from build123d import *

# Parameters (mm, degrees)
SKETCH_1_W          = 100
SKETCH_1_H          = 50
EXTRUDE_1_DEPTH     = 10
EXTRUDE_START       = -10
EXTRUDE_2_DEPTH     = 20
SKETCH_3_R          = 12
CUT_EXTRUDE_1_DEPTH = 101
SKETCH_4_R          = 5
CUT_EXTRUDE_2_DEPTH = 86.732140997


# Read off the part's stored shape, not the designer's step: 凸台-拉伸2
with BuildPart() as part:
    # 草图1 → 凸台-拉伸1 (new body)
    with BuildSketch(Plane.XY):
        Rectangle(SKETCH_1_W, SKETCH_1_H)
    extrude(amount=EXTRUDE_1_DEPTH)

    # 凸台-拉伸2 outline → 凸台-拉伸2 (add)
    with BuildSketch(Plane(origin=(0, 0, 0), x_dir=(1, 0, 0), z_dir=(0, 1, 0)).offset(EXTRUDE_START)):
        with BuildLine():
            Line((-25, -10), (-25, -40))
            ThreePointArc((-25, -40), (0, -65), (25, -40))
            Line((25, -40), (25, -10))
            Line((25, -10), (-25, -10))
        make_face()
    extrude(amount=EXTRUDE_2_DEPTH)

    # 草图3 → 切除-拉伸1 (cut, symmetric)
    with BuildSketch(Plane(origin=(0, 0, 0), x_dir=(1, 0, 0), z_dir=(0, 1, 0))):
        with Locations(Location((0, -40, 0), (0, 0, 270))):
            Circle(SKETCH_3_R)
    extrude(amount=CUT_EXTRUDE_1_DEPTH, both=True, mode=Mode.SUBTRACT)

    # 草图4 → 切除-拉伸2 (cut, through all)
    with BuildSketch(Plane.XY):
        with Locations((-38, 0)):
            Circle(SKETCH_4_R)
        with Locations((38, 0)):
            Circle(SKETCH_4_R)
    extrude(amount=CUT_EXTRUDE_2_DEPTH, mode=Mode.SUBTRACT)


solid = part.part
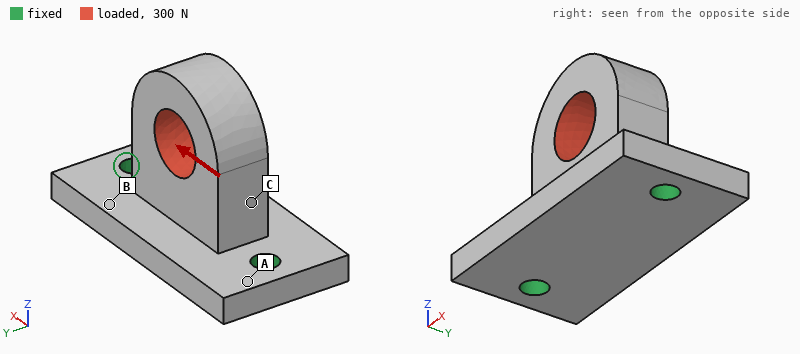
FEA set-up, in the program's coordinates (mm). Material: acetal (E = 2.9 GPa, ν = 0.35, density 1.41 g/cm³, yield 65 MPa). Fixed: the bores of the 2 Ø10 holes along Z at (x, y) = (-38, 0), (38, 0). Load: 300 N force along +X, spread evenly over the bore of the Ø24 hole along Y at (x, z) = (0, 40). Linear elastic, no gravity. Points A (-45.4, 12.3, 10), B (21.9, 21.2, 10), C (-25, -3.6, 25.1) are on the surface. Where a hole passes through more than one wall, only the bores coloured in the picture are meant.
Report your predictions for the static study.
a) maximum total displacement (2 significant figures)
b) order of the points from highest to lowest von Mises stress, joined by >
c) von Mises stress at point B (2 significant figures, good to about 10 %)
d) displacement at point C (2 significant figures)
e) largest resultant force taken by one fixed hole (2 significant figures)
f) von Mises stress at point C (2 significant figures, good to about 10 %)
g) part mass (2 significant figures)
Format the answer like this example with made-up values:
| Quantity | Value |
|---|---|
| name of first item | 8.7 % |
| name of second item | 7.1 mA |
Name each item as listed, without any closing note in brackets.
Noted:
| Quantity | Value |
|---|---|
| maximum total displacement | 67 µm |
| order of the points from highest to lowest von Mises stress, joined by > | C > B > A |
| von Mises stress at point B | 0.60 MPa |
| displacement at point C | 28 µm |
| largest resultant force taken by one fixed hole | 230 N |
| von Mises stress at point C | 1.1 MPa |
| part mass | 130 g |
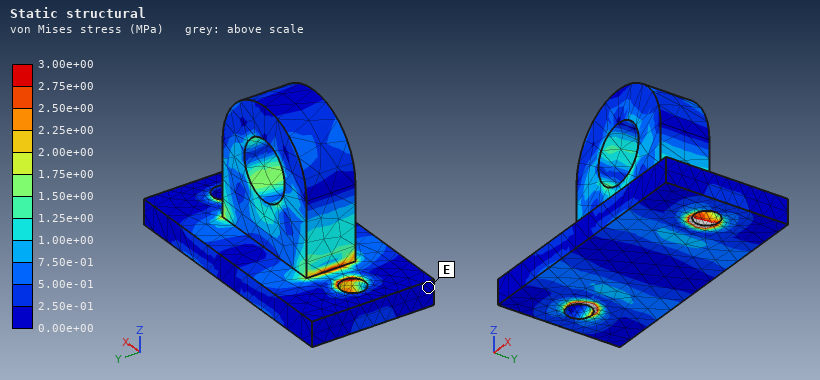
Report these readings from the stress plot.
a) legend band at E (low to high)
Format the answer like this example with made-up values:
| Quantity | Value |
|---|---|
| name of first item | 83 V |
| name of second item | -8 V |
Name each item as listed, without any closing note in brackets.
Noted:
| Quantity | Value |
|---|---|
| legend band at E | 0.00e+00 to 2.50e-01 MPa |
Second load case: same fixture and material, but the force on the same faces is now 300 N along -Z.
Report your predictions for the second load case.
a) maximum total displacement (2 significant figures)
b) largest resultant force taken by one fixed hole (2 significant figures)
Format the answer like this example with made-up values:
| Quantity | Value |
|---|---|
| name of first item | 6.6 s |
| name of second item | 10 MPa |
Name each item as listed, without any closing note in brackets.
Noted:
| Quantity | Value |
|---|---|
| maximum total displacement | 24 µm |
| largest resultant force taken by one fixed hole | 160 N |
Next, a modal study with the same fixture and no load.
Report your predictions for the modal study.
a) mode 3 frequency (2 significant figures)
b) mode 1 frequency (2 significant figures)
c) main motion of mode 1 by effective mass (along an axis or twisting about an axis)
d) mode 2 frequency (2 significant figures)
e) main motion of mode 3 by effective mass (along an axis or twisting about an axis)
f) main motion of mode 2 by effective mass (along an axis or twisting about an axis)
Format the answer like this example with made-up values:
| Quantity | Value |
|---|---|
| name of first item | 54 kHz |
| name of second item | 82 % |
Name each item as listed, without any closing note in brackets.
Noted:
| Quantity | Value |
|---|---|
| mode 3 frequency | 2100 Hz |
| mode 1 frequency | 730 Hz |
| main motion of mode 1 by effective mass | along Y |
| mode 2 frequency | 1800 Hz |
| main motion of mode 3 by effective mass | along Z |
| main motion of mode 2 by effective mass | along X |
